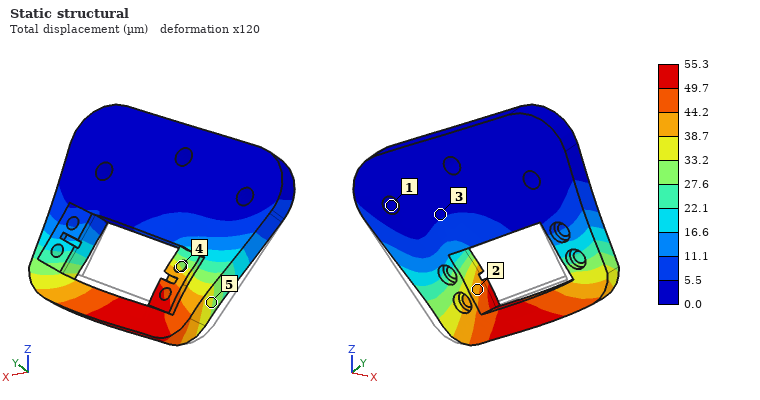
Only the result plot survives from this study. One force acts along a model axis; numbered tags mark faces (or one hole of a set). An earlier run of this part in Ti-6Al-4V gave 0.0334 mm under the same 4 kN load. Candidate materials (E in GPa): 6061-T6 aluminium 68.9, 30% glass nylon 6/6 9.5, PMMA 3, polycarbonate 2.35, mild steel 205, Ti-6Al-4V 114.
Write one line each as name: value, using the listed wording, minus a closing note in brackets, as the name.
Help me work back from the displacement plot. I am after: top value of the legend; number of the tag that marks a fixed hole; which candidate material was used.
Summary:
top value of the legend: 55.3 µm
number of the tag that marks a fixed hole: 1
which candidate material was used: 6061-T6 aluminium
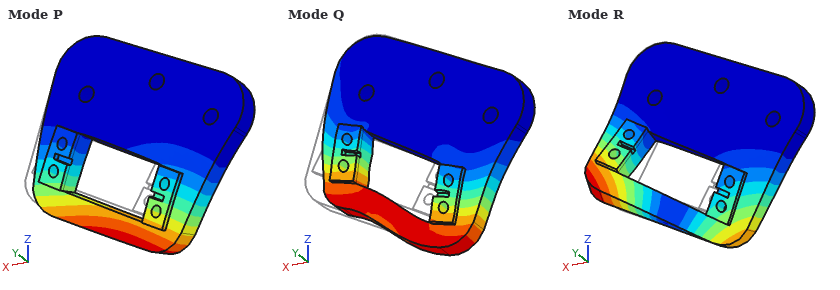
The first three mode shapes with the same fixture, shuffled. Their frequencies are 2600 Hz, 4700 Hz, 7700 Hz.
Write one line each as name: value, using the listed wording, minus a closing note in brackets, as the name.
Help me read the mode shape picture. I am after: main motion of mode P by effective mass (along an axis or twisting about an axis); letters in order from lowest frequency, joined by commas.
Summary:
main motion of mode P by effective mass: along Y
letters in order from lowest frequency, joined by commas: P, R, Q
